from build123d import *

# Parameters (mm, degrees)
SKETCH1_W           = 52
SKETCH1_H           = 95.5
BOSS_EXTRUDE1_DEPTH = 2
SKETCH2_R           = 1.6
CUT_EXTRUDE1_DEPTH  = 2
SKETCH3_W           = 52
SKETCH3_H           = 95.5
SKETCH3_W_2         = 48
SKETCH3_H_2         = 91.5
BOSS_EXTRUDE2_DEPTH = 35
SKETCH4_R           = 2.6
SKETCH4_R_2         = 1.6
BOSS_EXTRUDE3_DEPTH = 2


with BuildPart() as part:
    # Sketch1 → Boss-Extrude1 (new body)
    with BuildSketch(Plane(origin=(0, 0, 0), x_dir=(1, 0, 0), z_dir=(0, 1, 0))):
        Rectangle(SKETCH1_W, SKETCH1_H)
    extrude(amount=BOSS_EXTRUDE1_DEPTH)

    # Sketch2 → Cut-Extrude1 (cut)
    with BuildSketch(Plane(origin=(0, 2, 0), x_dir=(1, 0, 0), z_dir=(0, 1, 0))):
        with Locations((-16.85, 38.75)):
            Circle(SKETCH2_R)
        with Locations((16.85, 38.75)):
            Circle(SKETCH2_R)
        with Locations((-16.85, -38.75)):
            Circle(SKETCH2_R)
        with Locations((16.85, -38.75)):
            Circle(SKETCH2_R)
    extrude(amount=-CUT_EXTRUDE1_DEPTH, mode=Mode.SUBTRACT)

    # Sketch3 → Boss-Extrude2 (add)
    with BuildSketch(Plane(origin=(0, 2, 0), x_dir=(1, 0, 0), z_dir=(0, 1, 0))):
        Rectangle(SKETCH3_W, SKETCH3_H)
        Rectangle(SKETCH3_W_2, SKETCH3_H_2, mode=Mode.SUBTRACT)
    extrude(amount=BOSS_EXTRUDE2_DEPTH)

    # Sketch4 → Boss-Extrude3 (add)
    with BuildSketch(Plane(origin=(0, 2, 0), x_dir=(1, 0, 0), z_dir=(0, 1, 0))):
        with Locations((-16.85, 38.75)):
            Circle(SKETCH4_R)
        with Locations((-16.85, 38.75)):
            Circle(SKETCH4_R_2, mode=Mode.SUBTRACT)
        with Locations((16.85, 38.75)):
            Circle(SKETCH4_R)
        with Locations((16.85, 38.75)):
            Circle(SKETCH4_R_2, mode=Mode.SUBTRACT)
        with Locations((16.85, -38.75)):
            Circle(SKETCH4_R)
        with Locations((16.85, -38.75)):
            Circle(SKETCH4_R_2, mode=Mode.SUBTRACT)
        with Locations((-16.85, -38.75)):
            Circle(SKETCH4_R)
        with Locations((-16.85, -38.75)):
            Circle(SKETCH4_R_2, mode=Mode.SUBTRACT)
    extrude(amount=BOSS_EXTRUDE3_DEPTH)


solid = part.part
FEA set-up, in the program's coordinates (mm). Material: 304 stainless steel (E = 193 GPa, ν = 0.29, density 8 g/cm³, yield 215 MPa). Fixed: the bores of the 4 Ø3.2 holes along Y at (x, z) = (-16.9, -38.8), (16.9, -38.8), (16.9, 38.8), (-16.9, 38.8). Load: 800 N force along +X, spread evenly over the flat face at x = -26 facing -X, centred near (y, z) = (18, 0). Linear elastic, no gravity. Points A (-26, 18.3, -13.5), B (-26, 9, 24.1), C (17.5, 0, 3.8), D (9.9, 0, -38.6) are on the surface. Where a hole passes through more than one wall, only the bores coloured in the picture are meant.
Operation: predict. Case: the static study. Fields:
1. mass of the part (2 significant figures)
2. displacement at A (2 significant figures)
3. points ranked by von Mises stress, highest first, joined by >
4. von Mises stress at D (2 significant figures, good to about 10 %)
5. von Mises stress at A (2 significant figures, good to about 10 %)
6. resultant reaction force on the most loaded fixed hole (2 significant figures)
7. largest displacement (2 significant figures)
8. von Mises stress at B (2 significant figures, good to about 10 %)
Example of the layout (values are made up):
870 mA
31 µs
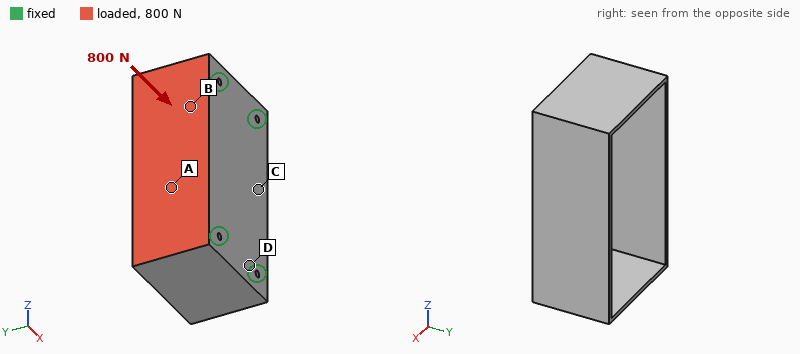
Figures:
240 g
0.11 mm
B > A > D > C
15 MPa
42 MPa
270 N
0.26 mm
52 MPa
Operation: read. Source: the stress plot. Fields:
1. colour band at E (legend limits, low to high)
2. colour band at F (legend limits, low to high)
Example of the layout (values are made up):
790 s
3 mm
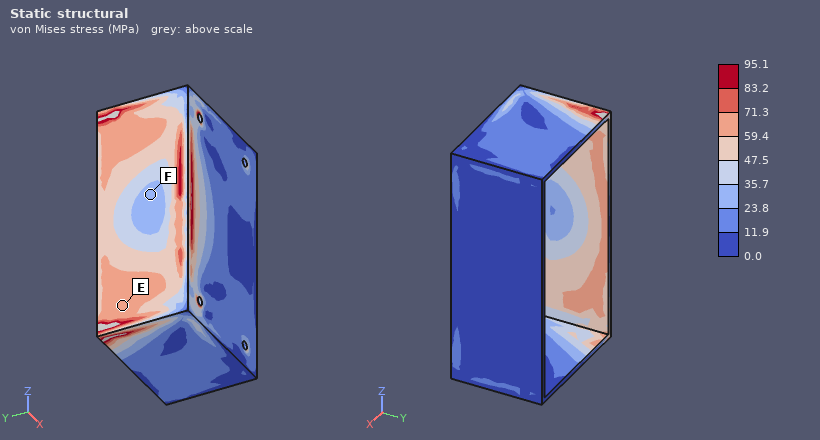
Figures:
59.4 to 71.3 MPa
23.8 to 35.7 MPa
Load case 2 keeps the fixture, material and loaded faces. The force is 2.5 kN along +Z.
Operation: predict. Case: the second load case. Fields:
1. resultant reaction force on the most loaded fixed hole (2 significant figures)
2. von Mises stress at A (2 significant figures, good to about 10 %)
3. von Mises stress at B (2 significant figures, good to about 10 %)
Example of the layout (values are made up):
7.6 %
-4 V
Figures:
1.2 kN
12 MPa
19 MPa
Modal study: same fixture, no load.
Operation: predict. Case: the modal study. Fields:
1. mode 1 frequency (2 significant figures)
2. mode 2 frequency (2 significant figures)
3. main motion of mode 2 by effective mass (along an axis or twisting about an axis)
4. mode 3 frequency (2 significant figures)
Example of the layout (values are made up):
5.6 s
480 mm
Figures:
1500 Hz
1600 Hz
along X
2900 Hz
